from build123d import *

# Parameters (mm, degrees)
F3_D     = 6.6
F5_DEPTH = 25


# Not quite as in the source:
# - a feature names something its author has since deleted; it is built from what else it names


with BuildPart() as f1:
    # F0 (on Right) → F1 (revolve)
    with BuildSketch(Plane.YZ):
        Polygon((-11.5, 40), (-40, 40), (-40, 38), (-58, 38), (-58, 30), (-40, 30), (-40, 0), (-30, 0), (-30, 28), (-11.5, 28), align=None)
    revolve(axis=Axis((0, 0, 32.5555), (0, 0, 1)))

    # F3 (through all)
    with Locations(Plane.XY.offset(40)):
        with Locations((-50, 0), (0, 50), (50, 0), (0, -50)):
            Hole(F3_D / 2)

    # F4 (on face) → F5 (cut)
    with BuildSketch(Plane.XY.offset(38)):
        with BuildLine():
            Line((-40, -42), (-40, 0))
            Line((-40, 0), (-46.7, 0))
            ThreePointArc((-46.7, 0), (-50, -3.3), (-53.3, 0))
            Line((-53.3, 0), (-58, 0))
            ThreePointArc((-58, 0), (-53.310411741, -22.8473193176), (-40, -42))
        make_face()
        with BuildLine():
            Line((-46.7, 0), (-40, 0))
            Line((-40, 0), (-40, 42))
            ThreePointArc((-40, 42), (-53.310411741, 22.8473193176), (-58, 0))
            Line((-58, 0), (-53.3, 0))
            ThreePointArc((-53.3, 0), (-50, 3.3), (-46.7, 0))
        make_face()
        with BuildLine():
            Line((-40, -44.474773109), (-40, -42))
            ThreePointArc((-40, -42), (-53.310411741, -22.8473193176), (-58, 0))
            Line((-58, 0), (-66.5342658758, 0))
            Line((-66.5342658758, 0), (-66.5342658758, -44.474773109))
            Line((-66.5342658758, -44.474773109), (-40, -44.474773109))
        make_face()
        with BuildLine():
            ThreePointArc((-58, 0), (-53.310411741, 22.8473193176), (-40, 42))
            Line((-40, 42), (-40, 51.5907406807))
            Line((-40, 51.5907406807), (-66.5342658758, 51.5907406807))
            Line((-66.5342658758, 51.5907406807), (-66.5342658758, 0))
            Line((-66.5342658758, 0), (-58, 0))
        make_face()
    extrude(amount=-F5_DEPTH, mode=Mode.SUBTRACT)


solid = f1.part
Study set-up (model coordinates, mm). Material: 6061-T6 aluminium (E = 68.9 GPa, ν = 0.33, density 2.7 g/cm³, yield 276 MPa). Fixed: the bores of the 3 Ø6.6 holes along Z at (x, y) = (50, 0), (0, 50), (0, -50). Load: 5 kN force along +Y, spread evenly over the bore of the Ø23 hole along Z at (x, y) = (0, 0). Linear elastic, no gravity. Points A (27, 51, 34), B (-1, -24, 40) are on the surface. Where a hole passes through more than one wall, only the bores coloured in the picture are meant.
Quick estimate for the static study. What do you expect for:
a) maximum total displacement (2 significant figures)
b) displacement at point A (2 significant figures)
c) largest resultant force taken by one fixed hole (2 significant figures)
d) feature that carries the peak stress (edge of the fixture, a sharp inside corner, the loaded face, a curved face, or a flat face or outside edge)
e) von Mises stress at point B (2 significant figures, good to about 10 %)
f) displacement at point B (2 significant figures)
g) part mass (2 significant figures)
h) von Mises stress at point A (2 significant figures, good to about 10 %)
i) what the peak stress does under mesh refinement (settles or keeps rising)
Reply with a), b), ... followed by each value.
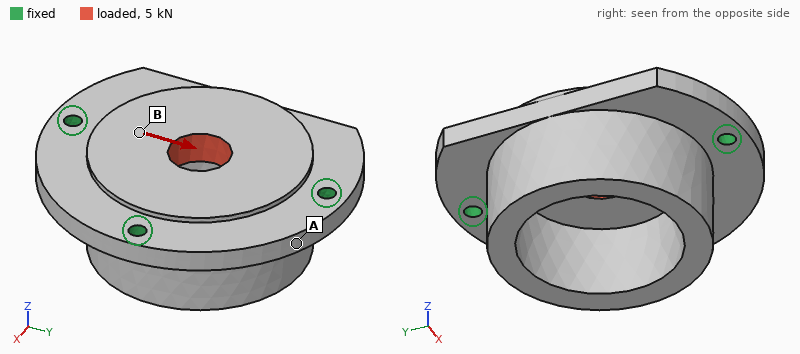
a) 5.3 µm
b) 2.4 µm
c) 2.1 kN
d) edge of the fixture
e) 7.0 MPa
f) 3.4 µm
g) 410 g
h) 3.1 MPa
i) keeps rising
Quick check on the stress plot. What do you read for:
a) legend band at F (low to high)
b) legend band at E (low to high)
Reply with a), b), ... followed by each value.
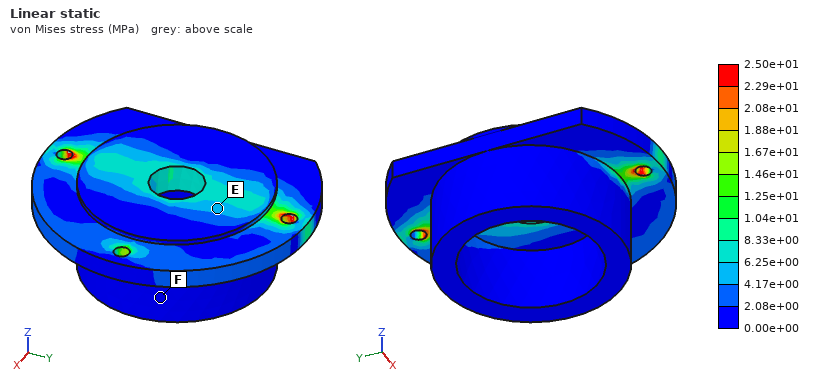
a) 0.00e+00 to 2.08e+00 MPa
b) 4.17e+00 to 6.25e+00 MPa
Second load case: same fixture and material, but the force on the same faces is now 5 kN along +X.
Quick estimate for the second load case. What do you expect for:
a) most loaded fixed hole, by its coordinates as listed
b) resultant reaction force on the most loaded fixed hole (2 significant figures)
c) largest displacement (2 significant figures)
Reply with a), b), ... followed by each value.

a) (50, 0)
b) 2.1 kN
c) 7.2 µm
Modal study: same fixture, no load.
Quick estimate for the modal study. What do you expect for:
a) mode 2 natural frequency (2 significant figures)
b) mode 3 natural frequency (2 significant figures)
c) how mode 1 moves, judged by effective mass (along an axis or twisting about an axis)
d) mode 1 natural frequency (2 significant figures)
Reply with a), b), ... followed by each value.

a) 6700 Hz
b) 6900 Hz
c) along Z
d) 2800 Hz
